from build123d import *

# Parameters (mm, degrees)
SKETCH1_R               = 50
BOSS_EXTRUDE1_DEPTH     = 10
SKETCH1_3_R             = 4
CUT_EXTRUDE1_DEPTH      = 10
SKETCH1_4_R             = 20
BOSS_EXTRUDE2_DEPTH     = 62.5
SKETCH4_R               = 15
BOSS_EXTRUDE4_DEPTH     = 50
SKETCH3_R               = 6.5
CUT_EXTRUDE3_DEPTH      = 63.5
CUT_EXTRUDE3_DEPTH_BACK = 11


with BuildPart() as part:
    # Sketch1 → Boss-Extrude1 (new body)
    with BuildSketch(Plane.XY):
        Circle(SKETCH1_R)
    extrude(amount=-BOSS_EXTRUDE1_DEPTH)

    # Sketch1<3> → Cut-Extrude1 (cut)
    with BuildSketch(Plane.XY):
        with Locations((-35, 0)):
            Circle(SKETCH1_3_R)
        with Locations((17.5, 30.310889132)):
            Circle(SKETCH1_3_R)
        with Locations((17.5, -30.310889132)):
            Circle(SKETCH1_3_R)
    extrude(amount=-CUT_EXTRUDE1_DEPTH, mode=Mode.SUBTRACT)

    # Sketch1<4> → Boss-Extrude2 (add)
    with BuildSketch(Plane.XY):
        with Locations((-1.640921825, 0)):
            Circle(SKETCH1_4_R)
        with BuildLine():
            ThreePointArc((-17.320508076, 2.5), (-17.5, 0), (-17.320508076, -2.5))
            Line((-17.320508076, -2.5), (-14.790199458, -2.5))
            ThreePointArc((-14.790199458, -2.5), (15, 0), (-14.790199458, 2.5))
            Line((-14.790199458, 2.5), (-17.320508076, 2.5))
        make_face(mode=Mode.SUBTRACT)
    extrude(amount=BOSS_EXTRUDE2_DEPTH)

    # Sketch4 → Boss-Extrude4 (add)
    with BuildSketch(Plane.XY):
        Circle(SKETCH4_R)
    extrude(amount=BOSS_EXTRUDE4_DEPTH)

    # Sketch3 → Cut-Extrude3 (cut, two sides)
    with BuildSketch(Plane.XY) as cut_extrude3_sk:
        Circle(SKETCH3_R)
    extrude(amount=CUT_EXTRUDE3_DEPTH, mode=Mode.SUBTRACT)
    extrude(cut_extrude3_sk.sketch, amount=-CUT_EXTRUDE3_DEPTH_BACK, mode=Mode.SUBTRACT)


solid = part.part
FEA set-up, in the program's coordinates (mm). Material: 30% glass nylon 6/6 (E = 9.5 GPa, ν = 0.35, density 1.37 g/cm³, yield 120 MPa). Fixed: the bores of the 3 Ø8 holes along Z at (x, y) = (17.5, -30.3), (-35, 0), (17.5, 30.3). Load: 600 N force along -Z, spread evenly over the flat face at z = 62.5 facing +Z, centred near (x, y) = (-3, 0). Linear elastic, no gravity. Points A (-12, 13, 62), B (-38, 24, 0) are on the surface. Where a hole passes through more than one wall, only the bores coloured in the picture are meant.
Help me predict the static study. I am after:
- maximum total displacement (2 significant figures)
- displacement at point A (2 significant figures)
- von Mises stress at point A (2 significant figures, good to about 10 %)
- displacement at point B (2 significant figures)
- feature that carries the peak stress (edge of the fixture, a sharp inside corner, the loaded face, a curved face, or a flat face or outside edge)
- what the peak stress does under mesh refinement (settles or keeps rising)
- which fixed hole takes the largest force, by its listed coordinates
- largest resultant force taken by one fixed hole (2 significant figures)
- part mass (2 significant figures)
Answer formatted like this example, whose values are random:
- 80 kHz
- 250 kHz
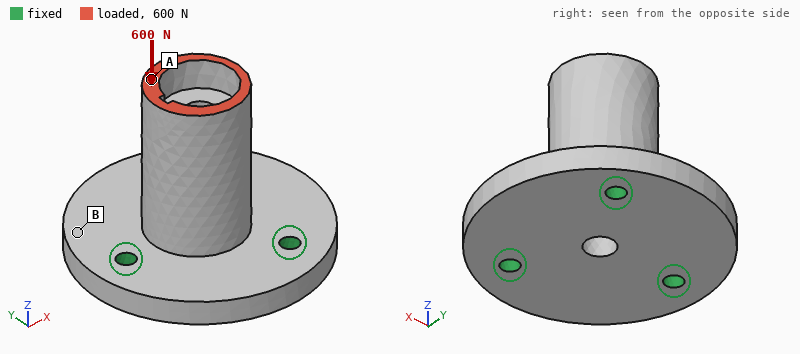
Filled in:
- 15 µm
- 14 µm
- 1.2 MPa
- 2.5 µm
- edge of the fixture
- keeps rising
- (-35, 0)
- 250 N
- 190 g
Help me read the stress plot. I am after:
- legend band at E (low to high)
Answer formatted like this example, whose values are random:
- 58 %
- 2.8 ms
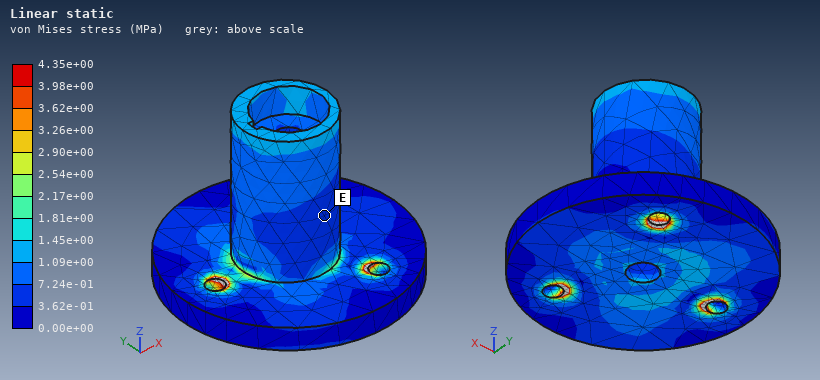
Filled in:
- 3.62e-01 to 7.24e-01 MPa
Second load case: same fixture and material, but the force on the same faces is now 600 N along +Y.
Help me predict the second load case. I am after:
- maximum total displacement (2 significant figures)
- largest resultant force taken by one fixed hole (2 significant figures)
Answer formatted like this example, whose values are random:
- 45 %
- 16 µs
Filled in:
- 0.18 mm
- 720 N
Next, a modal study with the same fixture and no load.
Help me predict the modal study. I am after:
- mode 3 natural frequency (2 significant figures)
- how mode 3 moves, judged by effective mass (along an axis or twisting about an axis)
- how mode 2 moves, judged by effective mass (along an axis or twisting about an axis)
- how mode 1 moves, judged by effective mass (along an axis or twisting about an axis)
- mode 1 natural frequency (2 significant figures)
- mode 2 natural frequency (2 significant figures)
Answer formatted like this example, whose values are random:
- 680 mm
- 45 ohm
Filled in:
- 3600 Hz
- along Z
- along X
- along Y
- 1900 Hz
- 2000 Hz
